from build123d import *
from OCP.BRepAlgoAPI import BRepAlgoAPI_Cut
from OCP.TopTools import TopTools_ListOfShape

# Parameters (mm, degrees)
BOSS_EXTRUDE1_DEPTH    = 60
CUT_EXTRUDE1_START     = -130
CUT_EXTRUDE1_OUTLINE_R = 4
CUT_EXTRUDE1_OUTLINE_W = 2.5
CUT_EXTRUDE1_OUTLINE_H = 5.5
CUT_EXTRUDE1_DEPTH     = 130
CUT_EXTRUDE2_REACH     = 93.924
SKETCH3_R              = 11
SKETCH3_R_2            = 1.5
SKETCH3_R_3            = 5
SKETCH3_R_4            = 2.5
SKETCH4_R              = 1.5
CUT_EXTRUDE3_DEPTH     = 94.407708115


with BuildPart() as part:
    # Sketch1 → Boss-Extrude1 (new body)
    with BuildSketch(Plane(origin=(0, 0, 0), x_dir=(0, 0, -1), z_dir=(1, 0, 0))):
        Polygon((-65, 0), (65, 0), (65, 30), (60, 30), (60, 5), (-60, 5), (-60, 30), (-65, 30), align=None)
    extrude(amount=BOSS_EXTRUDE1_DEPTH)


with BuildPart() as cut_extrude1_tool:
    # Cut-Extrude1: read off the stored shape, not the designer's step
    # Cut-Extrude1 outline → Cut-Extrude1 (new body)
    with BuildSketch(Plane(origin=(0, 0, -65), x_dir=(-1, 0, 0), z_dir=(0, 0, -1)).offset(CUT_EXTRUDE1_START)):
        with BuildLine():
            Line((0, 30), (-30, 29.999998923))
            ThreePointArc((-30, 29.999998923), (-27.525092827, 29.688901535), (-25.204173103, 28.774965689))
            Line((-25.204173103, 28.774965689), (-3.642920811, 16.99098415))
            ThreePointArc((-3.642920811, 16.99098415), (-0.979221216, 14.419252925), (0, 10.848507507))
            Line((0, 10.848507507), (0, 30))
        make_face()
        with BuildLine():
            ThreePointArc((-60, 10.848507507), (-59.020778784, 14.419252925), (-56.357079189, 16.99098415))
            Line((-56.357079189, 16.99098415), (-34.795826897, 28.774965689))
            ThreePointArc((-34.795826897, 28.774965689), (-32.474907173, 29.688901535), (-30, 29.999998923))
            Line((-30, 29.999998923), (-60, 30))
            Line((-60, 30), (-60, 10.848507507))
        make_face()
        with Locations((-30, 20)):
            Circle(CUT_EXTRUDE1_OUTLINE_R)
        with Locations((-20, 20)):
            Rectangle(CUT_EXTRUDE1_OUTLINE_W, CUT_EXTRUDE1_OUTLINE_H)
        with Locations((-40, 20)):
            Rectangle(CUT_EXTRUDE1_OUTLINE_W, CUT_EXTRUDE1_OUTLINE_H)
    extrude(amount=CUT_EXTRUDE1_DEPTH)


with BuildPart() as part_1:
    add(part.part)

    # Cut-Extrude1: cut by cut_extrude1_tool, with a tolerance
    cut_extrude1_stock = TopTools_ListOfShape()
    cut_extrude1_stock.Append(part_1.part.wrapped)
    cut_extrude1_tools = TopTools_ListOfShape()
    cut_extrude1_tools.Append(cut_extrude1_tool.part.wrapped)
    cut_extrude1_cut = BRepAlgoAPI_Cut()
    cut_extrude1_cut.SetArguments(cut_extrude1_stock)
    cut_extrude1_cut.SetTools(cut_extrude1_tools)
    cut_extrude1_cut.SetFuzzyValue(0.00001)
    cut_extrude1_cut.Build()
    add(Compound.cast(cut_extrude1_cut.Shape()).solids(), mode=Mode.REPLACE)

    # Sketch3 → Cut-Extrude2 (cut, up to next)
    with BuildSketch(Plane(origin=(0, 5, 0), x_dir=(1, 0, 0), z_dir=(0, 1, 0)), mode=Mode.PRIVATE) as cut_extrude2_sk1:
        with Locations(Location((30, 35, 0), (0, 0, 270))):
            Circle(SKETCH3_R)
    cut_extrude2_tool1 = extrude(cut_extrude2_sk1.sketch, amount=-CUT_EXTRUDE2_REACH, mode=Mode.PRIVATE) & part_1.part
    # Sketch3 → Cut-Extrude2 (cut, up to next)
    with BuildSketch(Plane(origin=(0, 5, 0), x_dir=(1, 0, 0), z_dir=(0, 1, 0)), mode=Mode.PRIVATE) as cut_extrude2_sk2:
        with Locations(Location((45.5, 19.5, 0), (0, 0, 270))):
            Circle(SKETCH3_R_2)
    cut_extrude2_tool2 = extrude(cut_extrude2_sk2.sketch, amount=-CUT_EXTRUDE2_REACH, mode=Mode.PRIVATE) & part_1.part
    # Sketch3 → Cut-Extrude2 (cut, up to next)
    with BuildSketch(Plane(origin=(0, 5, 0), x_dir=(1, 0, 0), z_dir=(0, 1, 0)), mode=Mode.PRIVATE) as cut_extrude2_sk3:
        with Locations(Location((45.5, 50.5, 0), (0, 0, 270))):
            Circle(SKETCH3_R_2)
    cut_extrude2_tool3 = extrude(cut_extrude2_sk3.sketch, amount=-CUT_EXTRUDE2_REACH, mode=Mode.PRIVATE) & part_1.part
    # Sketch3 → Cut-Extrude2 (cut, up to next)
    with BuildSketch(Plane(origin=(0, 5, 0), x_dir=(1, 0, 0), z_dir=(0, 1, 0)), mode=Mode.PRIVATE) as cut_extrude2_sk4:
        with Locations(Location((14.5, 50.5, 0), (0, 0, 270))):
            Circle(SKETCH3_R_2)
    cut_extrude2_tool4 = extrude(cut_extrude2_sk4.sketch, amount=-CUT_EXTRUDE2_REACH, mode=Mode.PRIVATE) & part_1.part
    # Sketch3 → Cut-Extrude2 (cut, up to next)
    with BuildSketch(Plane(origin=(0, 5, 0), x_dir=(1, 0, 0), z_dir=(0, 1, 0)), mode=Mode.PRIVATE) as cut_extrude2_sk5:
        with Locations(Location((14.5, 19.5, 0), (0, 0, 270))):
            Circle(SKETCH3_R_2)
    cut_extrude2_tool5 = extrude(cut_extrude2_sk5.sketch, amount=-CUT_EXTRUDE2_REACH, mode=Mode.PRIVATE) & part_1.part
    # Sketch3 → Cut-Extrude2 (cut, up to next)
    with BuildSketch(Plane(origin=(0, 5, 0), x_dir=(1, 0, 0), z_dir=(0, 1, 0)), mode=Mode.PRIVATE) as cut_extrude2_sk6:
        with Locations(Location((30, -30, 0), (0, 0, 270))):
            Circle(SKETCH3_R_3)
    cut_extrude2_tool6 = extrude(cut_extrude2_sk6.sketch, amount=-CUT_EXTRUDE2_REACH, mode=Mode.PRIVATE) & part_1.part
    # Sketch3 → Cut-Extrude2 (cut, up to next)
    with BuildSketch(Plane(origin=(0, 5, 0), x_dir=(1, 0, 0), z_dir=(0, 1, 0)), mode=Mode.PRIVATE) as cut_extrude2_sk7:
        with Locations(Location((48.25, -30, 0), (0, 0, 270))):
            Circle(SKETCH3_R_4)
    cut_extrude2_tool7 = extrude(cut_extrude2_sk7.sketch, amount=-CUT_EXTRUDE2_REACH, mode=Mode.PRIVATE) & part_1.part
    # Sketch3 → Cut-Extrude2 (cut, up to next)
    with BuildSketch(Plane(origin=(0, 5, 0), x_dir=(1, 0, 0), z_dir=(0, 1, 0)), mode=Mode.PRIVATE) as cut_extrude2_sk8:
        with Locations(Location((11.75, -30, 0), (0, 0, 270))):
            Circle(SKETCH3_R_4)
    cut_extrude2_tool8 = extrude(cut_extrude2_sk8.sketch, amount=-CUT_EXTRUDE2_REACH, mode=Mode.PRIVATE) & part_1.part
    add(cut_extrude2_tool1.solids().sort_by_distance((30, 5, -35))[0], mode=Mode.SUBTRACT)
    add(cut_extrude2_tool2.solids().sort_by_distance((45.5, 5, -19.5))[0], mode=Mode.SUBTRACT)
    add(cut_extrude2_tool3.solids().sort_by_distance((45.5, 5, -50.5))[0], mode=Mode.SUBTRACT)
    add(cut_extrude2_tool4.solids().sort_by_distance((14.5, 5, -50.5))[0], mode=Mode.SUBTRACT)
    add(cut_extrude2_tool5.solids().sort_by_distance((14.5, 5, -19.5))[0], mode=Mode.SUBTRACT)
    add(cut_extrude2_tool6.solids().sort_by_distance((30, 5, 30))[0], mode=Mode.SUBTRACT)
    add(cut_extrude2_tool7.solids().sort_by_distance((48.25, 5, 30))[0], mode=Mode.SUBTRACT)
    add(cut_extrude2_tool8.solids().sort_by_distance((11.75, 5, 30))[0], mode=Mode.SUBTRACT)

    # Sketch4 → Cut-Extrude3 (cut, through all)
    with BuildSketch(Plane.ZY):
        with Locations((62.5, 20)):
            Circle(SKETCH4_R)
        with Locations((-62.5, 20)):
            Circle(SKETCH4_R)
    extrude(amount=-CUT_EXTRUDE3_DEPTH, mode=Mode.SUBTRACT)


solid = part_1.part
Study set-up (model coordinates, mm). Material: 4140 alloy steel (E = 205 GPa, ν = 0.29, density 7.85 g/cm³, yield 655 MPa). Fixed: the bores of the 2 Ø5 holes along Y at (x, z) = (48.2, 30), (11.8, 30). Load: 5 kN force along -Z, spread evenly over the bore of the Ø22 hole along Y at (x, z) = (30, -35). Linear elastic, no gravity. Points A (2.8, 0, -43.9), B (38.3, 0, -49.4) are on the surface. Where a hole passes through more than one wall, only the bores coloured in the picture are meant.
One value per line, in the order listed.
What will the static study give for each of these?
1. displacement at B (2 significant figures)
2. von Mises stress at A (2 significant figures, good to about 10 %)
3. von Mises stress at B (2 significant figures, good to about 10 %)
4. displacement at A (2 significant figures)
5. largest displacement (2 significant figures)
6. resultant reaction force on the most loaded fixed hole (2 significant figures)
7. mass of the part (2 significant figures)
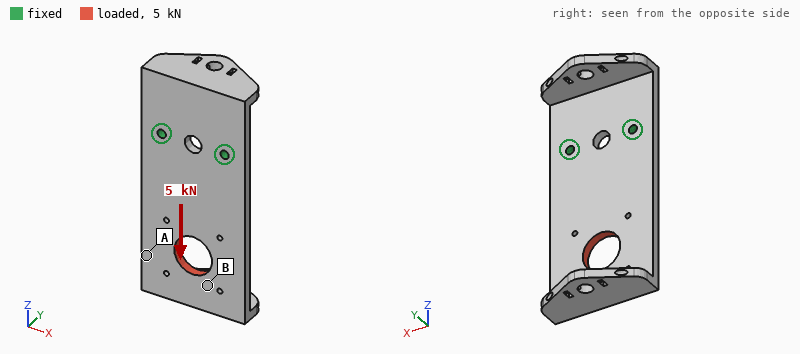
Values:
8.1 µm
5.2 MPa
14 MPa
5.8 µm
9.1 µm
2.5 kN
360 g
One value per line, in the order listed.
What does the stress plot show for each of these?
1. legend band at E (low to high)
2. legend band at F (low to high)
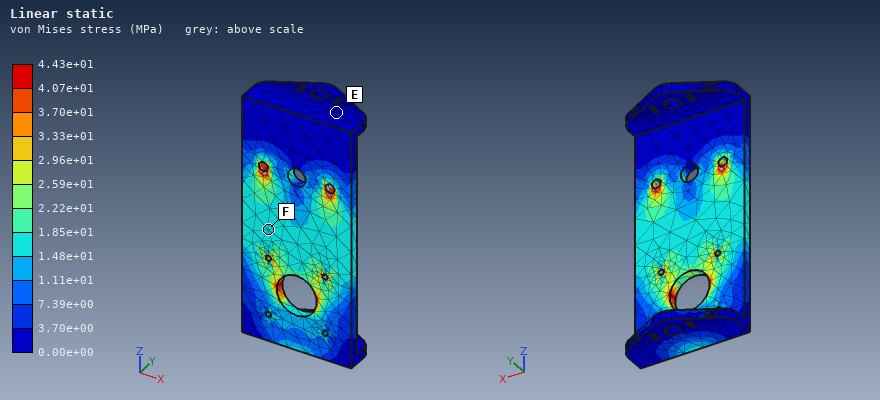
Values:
0.00e+00 to 3.70e+00 MPa
1.48e+01 to 1.85e+01 MPa
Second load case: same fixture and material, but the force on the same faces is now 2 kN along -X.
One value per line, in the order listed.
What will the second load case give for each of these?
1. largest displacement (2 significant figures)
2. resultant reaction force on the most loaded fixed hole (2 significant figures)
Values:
32 µm
3.5 kN
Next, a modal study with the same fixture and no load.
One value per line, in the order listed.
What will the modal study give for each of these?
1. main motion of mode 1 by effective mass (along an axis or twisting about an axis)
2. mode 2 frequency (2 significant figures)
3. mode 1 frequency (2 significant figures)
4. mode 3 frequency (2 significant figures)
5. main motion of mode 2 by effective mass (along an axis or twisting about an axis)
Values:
along Y
1200 Hz
350 Hz
1800 Hz
twisting about Z
